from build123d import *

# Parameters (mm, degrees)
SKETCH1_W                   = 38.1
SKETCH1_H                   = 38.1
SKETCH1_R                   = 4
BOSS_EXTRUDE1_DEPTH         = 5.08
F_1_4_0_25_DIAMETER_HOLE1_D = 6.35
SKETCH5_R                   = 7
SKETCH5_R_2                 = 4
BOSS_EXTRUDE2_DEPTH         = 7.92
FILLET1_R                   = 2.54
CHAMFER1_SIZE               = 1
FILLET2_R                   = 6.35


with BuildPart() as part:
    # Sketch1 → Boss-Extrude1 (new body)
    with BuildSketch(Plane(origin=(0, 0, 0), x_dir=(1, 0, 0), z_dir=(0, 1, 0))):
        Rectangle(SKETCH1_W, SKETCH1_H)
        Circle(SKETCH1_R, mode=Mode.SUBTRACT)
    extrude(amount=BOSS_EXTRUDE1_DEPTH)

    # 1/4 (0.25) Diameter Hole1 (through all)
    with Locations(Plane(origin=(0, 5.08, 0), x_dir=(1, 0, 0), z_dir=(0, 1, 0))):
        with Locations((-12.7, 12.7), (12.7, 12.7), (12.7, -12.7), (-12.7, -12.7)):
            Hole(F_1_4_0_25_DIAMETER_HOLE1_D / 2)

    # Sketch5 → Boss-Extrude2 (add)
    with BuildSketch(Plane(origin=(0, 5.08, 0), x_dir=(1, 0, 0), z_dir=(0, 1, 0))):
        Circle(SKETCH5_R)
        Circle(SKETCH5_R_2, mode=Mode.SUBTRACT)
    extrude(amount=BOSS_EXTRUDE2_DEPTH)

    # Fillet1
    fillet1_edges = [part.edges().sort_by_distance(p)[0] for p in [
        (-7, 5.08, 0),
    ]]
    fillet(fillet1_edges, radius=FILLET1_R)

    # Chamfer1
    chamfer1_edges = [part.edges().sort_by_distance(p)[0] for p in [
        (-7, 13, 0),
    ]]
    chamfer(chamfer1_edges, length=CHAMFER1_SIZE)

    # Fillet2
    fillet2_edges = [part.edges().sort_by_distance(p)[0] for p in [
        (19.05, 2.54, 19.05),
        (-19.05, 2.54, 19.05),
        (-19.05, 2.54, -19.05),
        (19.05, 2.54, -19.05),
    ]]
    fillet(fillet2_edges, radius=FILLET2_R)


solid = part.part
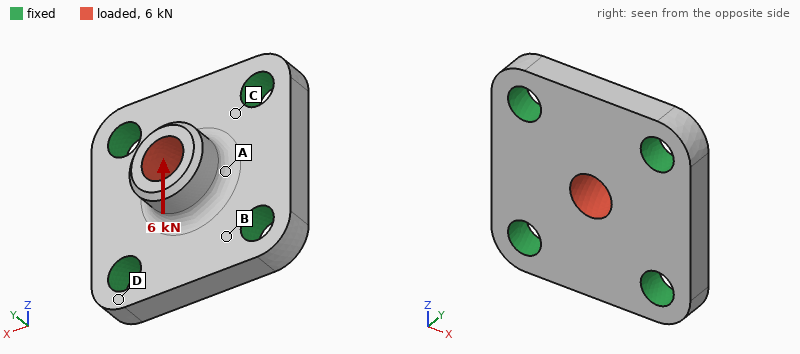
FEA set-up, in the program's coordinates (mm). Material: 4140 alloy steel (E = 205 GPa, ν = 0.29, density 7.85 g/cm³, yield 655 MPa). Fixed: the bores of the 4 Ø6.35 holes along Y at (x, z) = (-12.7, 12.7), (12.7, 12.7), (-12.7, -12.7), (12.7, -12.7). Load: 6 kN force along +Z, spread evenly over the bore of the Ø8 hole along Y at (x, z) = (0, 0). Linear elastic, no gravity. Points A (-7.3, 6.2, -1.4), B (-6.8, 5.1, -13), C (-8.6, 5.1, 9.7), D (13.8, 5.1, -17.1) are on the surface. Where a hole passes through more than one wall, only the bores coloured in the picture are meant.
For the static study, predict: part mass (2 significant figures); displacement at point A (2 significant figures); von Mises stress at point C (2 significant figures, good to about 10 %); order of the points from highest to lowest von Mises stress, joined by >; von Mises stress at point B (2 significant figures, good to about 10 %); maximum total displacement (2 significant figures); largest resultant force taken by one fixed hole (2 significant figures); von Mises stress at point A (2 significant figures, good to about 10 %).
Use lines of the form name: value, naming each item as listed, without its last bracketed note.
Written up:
part mass: 56 g
displacement at point A: 2.7 µm
von Mises stress at point C: 35 MPa
order of the points from highest to lowest von Mises stress, joined by >: A > C > B > D
von Mises stress at point B: 19 MPa
maximum total displacement: 8.6 µm
largest resultant force taken by one fixed hole: 1.7 kN
von Mises stress at point A: 76 MPa
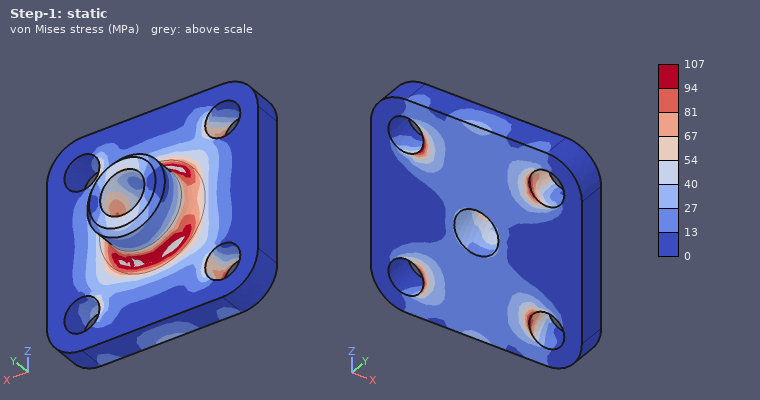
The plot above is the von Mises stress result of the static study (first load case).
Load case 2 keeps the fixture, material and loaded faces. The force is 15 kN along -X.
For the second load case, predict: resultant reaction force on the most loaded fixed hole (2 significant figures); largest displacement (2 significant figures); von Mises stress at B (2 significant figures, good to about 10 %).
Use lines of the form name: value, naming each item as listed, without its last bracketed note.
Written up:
resultant reaction force on the most loaded fixed hole: 4.4 kN
largest displacement: 22 µm
von Mises stress at B: 50 MPa
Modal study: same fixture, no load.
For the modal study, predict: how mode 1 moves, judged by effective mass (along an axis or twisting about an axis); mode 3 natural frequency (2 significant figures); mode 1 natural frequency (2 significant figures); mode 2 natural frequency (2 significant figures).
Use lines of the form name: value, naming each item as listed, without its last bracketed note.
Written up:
how mode 1 moves, judged by effective mass: along Y
mode 3 natural frequency: 40 kHz
mode 1 natural frequency: 31 kHz
mode 2 natural frequency: 40 kHz
